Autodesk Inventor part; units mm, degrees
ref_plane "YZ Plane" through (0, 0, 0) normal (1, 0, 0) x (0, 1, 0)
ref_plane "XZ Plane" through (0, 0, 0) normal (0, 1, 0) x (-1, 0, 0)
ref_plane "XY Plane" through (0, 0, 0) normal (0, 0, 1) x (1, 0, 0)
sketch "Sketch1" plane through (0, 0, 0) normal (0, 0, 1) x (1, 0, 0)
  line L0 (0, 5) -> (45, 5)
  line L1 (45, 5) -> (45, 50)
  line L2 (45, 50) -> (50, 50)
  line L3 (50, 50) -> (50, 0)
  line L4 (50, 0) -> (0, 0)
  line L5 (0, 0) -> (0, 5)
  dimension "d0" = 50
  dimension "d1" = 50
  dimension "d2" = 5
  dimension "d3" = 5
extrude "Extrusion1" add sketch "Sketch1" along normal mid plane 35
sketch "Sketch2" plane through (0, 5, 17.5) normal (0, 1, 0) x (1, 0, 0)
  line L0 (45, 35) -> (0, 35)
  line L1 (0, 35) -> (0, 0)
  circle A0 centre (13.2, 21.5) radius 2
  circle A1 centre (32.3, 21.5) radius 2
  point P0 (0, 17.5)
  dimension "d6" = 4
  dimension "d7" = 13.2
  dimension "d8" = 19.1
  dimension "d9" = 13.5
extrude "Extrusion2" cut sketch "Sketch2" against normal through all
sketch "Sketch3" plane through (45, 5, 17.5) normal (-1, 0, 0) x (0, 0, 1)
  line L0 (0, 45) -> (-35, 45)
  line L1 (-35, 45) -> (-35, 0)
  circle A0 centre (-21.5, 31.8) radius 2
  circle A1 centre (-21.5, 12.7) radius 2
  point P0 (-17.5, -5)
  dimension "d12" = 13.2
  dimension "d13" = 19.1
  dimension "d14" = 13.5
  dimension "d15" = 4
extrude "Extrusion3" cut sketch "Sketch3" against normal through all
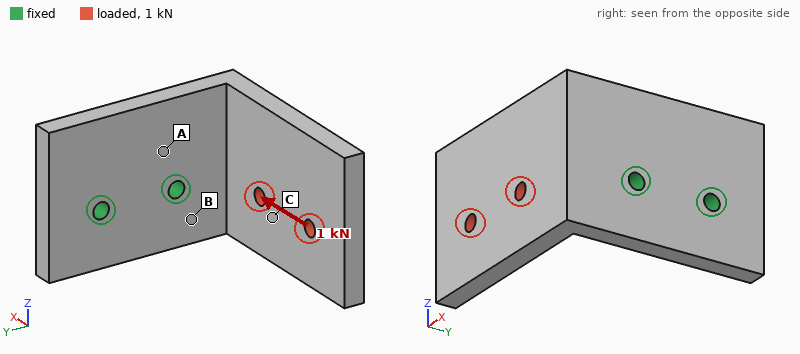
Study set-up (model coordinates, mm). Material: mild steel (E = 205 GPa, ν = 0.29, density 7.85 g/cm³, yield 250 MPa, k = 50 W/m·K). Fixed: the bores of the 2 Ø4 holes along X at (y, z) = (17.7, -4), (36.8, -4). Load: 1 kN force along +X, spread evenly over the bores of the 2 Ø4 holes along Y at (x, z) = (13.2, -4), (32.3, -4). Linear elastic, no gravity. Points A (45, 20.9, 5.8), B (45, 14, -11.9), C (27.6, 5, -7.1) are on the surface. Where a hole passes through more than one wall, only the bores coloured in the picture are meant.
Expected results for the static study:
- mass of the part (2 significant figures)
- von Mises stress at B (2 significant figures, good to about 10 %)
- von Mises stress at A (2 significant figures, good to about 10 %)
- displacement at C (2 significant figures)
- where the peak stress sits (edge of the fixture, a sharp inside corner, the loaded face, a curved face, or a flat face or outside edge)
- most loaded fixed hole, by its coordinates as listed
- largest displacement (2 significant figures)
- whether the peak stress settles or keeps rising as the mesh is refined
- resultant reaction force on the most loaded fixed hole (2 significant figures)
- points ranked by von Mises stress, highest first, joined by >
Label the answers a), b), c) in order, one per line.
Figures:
a) 130 g
b) 66 MPa
c) 37 MPa
d) 42 µm
e) edge of the fixture
f) (17.7, -4)
g) 95 µm
h) keeps rising
i) 1.3 kN
j) B > A > C
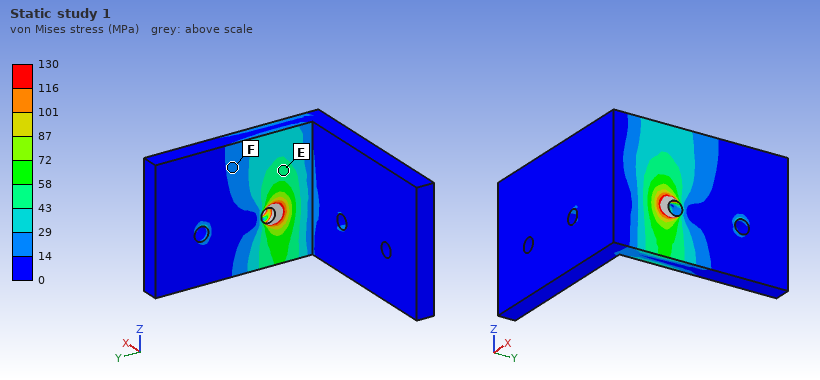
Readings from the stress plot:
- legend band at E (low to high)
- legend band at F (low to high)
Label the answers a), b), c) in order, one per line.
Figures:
a) 43 to 58 MPa
b) 14 to 29 MPa
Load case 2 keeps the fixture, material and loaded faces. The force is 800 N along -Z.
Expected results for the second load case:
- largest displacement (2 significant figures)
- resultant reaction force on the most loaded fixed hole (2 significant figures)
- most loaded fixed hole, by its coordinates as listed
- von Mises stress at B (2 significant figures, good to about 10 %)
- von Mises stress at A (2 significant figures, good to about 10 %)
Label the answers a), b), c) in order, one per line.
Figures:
a) 0.15 mm
b) 1.3 kN
c) (17.7, -4)
d) 81 MPa
e) 61 MPa
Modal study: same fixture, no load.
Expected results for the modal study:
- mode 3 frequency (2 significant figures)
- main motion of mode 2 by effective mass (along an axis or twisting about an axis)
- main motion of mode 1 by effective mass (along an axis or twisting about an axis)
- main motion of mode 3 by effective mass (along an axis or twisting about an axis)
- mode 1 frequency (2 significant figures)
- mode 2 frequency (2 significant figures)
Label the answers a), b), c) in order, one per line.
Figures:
a) 4900 Hz
b) along Z
c) along Y
d) along X
e) 1200 Hz
f) 1800 Hz
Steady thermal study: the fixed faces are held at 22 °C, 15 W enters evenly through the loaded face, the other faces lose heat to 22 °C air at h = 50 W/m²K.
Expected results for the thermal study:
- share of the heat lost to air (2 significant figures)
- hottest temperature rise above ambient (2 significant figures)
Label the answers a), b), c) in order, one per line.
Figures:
a) 49 %
b) 47 K
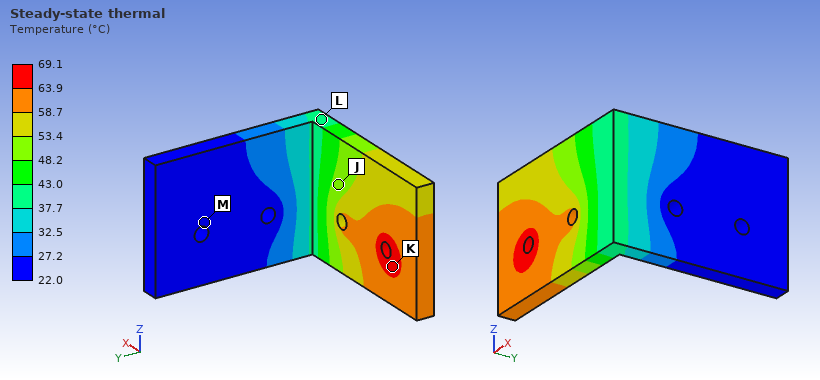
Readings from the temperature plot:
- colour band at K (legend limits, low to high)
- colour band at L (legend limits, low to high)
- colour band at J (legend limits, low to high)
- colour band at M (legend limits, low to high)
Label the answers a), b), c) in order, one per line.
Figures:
a) 63.9 to 69.1 °C
b) 37.7 to 43.0 °C
c) 48.2 to 53.4 °C
d) 22.0 to 27.2 °C
